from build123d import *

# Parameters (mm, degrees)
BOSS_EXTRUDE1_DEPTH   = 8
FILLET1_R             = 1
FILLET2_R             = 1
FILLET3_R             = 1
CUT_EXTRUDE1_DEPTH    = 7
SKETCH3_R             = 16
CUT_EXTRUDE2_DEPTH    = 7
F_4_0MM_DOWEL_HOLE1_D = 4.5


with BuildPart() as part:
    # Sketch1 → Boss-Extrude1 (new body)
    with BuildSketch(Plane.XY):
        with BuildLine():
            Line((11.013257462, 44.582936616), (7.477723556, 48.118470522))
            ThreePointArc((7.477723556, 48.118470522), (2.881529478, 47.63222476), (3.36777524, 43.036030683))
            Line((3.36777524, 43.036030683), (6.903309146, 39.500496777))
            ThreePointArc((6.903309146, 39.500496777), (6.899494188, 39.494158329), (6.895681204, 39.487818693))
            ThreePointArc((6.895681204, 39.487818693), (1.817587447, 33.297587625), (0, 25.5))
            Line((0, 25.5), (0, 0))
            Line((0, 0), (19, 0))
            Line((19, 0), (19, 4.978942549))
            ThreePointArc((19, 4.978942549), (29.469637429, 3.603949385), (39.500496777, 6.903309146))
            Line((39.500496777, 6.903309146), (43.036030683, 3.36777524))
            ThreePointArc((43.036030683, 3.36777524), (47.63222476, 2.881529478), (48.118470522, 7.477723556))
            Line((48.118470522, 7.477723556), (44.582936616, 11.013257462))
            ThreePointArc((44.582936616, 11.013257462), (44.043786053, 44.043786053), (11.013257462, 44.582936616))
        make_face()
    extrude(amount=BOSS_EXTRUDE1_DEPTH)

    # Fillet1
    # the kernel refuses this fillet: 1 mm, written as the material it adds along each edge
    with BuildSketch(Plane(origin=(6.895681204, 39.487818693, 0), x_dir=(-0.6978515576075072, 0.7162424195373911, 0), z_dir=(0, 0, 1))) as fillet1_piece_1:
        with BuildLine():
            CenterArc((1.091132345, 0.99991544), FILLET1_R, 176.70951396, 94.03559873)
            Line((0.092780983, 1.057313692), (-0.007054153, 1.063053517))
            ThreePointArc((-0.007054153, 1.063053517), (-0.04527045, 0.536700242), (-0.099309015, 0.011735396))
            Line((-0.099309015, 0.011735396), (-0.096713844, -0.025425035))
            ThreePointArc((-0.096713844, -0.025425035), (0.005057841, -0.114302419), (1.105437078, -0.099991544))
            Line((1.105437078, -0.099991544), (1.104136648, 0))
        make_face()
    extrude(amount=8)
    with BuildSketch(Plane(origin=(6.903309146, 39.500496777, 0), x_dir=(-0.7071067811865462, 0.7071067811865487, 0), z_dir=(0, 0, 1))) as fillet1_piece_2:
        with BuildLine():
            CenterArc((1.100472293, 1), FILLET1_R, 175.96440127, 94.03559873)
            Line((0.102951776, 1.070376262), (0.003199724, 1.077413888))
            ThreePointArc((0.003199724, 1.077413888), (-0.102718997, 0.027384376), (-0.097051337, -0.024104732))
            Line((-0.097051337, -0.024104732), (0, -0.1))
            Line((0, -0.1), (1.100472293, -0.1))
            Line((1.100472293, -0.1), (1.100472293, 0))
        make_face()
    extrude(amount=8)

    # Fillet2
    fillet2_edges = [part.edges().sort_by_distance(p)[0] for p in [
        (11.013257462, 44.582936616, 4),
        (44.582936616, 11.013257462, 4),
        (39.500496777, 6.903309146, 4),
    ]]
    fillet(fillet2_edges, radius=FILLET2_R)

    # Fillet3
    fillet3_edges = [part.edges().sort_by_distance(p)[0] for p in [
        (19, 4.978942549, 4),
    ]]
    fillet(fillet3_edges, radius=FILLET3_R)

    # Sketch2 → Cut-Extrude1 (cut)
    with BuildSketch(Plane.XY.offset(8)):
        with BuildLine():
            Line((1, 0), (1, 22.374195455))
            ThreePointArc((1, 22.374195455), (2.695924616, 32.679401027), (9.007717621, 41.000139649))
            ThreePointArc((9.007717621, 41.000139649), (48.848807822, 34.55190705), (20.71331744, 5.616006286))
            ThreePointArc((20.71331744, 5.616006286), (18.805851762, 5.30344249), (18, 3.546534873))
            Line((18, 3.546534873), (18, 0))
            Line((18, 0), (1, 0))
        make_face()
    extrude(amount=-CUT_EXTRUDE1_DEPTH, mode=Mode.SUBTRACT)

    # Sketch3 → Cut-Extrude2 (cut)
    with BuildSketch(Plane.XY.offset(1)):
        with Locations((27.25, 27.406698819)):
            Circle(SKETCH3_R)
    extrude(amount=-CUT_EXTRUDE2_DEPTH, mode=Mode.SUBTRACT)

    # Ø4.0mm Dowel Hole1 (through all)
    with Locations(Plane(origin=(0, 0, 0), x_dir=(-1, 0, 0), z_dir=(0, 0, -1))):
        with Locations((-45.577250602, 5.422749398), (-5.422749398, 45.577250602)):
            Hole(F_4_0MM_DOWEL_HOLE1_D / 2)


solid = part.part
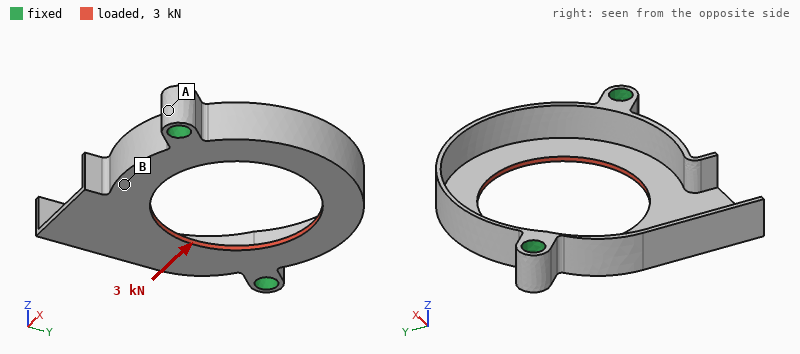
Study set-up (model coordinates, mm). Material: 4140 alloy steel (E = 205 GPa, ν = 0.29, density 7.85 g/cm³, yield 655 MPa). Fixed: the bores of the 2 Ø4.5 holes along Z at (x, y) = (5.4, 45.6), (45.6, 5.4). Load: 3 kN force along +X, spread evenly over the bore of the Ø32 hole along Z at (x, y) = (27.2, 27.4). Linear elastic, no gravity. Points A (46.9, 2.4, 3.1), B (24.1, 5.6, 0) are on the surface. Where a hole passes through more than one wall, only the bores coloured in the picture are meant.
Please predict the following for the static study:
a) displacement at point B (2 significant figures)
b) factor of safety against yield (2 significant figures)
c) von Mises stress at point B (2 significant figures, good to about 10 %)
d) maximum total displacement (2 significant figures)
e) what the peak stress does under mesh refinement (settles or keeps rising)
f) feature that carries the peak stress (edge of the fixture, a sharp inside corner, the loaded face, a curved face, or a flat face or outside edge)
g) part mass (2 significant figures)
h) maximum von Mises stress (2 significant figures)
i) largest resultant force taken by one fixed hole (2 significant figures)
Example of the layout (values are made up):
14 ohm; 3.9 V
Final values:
29 µm; 0.88; 56 MPa; 62 µm; settles; a curved face; 22 g; 740 MPa; 1.5 kN
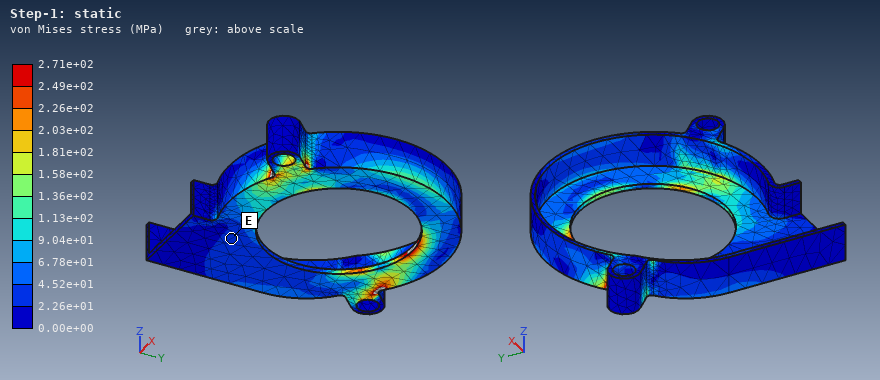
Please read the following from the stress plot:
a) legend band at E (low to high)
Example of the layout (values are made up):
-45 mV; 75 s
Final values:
2.26e+01 to 4.52e+01 MPa
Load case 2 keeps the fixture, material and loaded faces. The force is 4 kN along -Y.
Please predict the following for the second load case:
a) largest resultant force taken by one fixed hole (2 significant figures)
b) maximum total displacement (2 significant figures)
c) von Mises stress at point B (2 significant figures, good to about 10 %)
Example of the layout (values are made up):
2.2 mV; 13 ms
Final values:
2.1 kN; 80 µm; 92 MPa
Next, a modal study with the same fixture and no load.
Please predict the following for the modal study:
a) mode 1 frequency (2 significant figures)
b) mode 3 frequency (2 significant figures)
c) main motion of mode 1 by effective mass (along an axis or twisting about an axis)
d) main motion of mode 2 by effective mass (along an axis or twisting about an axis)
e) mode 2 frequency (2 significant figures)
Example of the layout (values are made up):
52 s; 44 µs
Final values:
2200 Hz; 4600 Hz; along Z; along Z; 3800 Hz
